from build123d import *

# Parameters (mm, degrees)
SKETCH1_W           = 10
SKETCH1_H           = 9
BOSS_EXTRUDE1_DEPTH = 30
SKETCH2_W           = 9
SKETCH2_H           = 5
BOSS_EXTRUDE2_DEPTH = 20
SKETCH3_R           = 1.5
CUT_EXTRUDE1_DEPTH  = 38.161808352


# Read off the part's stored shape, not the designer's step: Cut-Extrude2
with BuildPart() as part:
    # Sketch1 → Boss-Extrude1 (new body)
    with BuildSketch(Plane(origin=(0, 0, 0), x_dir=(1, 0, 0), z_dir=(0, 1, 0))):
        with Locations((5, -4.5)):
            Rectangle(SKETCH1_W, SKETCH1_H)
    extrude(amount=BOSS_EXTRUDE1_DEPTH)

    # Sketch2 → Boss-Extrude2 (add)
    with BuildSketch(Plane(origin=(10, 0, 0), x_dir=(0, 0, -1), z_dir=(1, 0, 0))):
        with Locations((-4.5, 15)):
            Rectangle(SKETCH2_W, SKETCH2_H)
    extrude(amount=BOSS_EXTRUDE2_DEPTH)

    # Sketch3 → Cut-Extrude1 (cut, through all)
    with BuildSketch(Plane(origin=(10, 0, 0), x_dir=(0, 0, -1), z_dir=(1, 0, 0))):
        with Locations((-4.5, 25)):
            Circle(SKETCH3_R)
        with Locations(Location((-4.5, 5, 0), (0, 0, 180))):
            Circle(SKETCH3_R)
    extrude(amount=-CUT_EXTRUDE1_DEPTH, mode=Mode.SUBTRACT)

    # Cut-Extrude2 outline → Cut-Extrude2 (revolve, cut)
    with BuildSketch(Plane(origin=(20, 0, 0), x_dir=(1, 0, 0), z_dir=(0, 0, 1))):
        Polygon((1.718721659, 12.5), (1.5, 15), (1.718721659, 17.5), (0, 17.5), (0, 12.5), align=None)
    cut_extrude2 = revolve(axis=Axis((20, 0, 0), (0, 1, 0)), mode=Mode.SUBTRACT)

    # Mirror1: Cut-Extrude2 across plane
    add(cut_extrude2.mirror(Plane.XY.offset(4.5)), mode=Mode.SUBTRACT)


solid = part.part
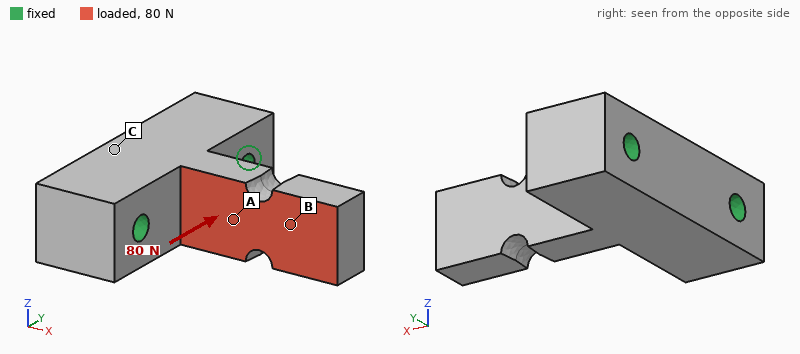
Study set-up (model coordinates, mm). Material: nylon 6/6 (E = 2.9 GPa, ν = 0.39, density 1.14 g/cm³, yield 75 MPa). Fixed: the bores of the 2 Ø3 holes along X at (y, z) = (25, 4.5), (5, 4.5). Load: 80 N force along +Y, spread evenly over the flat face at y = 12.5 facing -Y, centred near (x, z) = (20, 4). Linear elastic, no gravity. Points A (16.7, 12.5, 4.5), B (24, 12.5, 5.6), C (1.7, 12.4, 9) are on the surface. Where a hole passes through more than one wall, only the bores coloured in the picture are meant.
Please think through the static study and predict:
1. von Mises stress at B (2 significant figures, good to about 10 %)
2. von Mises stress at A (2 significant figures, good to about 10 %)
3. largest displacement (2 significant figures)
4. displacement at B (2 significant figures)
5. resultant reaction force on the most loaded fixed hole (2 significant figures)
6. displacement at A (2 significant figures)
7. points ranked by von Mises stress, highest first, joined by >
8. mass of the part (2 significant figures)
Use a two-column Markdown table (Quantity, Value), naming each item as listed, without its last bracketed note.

| Quantity | Value |
|---|---|
| von Mises stress at B | 2.6 MPa |
| von Mises stress at A | 12 MPa |
| largest displacement | 0.46 mm |
| displacement at B | 0.29 mm |
| resultant reaction force on the most loaded fixed hole | 79 N |
| displacement at A | 0.12 mm |
| points ranked by von Mises stress, highest first, joined by > | A > B > C |
| mass of the part | 3.9 g |
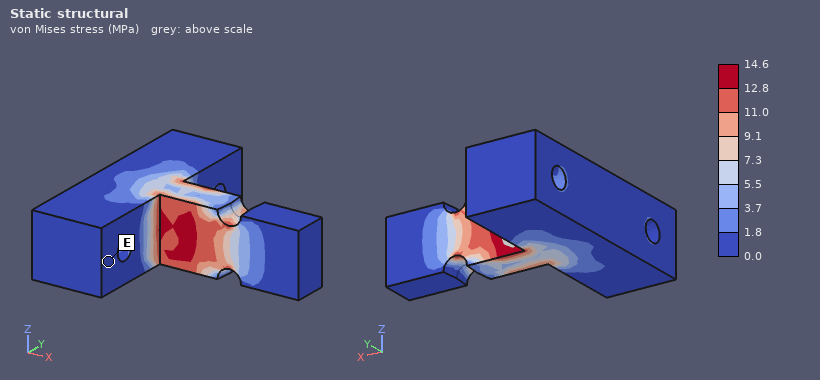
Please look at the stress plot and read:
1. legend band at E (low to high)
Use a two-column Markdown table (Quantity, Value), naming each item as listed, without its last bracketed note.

| Quantity | Value |
|---|---|
| legend band at E | 0.0 to 1.8 MPa |
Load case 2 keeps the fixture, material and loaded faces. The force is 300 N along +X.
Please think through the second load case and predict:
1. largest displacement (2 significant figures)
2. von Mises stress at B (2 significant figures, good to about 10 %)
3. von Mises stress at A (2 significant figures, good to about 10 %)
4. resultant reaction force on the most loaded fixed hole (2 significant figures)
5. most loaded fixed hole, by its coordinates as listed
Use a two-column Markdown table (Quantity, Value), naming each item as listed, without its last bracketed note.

| Quantity | Value |
|---|---|
| largest displacement | 0.52 mm |
| von Mises stress at B | 11 MPa |
| von Mises stress at A | 21 MPa |
| resultant reaction force on the most loaded fixed hole | 200 N |
| most loaded fixed hole, by its coordinates as listed | (5, 4.5) |
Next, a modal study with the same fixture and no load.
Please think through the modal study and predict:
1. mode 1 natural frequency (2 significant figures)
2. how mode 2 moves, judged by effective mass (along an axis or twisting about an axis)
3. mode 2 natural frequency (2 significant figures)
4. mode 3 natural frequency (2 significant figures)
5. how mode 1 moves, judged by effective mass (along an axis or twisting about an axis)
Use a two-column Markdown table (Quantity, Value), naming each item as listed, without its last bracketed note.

| Quantity | Value |
|---|---|
| mode 1 natural frequency | 2600 Hz |
| how mode 2 moves, judged by effective mass | along Z |
| mode 2 natural frequency | 3100 Hz |
| mode 3 natural frequency | 9000 Hz |
| how mode 1 moves, judged by effective mass | along Y |
